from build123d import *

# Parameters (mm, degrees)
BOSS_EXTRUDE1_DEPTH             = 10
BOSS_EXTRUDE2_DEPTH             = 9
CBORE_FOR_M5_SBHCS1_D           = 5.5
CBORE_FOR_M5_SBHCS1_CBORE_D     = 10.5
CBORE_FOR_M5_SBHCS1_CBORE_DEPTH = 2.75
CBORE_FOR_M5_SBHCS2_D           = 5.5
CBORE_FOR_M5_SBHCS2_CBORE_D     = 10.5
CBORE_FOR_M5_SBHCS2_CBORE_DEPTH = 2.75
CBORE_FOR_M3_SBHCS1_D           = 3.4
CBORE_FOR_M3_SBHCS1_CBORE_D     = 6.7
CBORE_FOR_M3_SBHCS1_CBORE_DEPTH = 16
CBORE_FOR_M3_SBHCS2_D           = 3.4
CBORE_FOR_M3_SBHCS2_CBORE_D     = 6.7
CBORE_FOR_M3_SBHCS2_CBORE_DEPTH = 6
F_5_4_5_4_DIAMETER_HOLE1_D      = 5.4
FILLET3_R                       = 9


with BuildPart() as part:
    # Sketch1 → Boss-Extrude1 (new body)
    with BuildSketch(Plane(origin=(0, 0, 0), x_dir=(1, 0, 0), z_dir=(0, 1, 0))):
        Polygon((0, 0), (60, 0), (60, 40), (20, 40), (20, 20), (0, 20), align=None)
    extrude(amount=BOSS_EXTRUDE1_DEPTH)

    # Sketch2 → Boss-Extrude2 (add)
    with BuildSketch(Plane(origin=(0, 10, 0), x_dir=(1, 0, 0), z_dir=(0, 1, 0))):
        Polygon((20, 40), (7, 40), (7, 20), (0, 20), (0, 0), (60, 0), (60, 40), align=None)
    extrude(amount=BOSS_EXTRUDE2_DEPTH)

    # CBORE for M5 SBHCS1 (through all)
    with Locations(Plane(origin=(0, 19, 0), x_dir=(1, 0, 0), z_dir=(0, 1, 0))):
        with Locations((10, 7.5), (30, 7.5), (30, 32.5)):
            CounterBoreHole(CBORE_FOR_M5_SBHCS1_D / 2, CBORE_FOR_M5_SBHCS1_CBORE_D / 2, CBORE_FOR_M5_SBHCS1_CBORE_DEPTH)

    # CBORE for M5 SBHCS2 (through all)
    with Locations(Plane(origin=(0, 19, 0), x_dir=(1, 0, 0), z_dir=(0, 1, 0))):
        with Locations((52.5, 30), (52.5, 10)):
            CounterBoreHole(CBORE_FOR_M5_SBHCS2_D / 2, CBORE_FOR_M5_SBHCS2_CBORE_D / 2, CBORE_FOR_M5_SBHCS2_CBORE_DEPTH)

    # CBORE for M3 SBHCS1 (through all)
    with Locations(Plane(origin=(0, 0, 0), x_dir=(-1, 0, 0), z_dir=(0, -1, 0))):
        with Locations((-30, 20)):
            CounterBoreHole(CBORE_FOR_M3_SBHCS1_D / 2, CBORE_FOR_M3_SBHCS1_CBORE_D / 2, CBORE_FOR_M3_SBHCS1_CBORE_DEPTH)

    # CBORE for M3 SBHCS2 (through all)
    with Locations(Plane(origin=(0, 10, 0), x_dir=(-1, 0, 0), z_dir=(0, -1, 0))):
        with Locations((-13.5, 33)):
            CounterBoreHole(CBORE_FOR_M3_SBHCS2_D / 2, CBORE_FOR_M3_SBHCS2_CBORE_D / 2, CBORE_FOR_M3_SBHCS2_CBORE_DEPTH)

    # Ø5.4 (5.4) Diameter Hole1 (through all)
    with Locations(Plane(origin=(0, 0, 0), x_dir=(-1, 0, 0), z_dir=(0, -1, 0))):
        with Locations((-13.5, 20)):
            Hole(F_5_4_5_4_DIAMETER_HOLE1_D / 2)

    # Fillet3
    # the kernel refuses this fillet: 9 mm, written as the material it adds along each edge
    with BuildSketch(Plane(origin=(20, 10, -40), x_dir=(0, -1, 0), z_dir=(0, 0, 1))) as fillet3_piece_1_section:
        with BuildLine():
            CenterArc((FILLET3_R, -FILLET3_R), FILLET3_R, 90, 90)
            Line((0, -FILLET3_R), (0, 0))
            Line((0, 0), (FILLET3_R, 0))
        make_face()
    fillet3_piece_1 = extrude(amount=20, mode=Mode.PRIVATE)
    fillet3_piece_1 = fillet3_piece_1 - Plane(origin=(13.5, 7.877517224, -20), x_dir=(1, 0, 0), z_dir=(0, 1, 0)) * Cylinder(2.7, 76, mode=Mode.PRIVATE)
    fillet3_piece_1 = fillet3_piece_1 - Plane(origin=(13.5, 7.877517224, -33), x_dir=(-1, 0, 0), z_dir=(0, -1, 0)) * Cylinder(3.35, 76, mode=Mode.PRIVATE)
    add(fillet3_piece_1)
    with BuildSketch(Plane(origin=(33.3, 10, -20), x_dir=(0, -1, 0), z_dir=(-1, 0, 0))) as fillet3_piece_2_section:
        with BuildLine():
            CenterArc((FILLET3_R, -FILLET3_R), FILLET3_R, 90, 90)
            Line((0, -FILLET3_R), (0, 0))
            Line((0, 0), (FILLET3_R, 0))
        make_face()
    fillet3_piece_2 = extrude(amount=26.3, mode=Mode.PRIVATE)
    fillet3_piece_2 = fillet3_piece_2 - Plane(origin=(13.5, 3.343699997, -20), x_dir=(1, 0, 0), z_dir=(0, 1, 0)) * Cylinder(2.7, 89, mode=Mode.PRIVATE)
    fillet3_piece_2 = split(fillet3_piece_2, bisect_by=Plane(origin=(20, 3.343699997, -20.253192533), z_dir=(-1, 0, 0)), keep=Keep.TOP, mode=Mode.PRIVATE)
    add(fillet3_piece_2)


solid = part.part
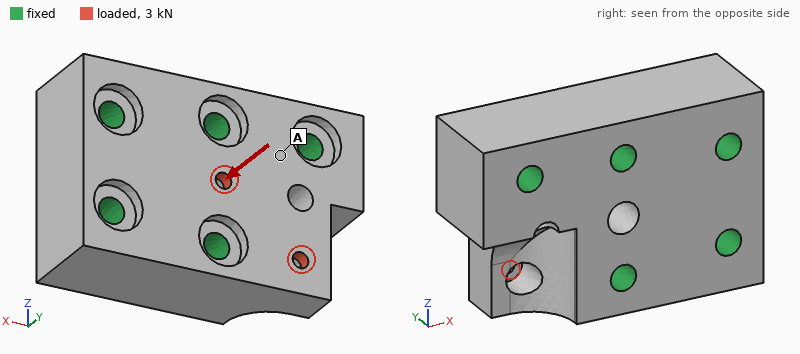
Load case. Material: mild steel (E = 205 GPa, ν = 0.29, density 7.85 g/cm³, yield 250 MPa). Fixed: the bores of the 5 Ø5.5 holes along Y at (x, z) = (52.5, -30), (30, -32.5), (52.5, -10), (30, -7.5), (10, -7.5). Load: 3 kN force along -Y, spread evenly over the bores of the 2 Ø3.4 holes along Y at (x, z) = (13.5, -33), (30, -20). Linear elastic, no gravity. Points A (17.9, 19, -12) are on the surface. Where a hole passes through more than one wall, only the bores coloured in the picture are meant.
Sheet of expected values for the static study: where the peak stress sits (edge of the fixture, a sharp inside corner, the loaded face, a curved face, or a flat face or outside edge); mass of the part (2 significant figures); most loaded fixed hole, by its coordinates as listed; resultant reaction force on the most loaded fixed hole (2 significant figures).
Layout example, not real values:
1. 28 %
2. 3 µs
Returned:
1. the loaded face
2. 290 g
3. (30, -32.5)
4. 1.9 kN
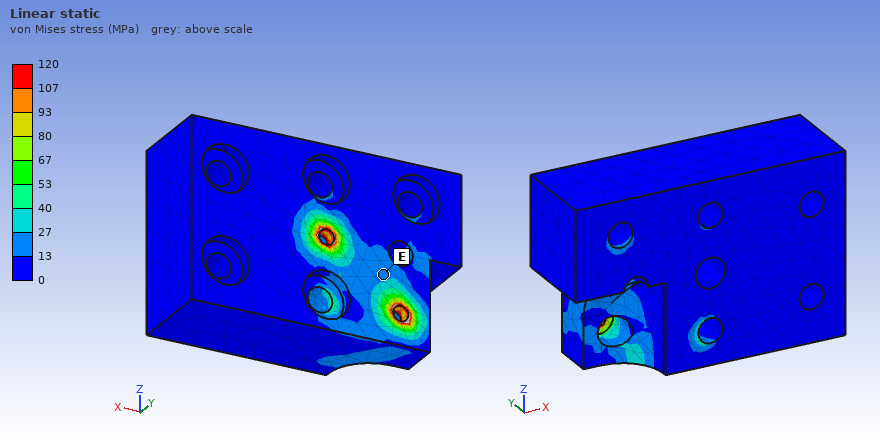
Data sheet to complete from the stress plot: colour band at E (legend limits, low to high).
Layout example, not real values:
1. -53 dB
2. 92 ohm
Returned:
1. 13 to 27 MPa
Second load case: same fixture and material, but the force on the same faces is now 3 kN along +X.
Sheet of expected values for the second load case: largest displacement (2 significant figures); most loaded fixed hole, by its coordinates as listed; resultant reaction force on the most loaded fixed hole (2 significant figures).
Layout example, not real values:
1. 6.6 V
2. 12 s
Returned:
1. 3.3 µm
2. (30, -32.5)
3. 1.5 kN
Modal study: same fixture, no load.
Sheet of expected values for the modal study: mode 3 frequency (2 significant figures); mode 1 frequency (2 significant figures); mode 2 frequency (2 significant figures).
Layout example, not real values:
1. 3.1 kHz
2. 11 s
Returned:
1. 47 kHz
2. 29 kHz
3. 44 kHz
